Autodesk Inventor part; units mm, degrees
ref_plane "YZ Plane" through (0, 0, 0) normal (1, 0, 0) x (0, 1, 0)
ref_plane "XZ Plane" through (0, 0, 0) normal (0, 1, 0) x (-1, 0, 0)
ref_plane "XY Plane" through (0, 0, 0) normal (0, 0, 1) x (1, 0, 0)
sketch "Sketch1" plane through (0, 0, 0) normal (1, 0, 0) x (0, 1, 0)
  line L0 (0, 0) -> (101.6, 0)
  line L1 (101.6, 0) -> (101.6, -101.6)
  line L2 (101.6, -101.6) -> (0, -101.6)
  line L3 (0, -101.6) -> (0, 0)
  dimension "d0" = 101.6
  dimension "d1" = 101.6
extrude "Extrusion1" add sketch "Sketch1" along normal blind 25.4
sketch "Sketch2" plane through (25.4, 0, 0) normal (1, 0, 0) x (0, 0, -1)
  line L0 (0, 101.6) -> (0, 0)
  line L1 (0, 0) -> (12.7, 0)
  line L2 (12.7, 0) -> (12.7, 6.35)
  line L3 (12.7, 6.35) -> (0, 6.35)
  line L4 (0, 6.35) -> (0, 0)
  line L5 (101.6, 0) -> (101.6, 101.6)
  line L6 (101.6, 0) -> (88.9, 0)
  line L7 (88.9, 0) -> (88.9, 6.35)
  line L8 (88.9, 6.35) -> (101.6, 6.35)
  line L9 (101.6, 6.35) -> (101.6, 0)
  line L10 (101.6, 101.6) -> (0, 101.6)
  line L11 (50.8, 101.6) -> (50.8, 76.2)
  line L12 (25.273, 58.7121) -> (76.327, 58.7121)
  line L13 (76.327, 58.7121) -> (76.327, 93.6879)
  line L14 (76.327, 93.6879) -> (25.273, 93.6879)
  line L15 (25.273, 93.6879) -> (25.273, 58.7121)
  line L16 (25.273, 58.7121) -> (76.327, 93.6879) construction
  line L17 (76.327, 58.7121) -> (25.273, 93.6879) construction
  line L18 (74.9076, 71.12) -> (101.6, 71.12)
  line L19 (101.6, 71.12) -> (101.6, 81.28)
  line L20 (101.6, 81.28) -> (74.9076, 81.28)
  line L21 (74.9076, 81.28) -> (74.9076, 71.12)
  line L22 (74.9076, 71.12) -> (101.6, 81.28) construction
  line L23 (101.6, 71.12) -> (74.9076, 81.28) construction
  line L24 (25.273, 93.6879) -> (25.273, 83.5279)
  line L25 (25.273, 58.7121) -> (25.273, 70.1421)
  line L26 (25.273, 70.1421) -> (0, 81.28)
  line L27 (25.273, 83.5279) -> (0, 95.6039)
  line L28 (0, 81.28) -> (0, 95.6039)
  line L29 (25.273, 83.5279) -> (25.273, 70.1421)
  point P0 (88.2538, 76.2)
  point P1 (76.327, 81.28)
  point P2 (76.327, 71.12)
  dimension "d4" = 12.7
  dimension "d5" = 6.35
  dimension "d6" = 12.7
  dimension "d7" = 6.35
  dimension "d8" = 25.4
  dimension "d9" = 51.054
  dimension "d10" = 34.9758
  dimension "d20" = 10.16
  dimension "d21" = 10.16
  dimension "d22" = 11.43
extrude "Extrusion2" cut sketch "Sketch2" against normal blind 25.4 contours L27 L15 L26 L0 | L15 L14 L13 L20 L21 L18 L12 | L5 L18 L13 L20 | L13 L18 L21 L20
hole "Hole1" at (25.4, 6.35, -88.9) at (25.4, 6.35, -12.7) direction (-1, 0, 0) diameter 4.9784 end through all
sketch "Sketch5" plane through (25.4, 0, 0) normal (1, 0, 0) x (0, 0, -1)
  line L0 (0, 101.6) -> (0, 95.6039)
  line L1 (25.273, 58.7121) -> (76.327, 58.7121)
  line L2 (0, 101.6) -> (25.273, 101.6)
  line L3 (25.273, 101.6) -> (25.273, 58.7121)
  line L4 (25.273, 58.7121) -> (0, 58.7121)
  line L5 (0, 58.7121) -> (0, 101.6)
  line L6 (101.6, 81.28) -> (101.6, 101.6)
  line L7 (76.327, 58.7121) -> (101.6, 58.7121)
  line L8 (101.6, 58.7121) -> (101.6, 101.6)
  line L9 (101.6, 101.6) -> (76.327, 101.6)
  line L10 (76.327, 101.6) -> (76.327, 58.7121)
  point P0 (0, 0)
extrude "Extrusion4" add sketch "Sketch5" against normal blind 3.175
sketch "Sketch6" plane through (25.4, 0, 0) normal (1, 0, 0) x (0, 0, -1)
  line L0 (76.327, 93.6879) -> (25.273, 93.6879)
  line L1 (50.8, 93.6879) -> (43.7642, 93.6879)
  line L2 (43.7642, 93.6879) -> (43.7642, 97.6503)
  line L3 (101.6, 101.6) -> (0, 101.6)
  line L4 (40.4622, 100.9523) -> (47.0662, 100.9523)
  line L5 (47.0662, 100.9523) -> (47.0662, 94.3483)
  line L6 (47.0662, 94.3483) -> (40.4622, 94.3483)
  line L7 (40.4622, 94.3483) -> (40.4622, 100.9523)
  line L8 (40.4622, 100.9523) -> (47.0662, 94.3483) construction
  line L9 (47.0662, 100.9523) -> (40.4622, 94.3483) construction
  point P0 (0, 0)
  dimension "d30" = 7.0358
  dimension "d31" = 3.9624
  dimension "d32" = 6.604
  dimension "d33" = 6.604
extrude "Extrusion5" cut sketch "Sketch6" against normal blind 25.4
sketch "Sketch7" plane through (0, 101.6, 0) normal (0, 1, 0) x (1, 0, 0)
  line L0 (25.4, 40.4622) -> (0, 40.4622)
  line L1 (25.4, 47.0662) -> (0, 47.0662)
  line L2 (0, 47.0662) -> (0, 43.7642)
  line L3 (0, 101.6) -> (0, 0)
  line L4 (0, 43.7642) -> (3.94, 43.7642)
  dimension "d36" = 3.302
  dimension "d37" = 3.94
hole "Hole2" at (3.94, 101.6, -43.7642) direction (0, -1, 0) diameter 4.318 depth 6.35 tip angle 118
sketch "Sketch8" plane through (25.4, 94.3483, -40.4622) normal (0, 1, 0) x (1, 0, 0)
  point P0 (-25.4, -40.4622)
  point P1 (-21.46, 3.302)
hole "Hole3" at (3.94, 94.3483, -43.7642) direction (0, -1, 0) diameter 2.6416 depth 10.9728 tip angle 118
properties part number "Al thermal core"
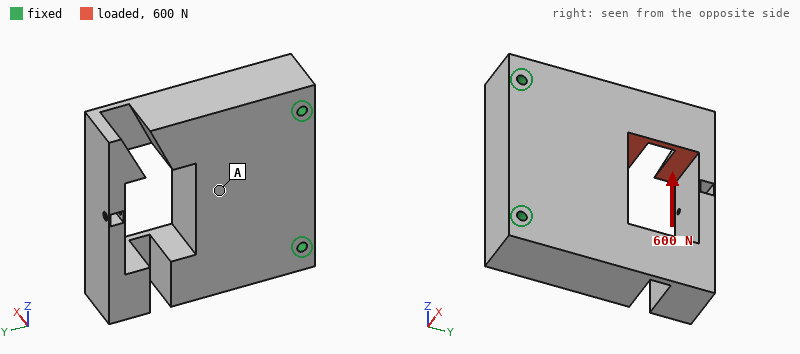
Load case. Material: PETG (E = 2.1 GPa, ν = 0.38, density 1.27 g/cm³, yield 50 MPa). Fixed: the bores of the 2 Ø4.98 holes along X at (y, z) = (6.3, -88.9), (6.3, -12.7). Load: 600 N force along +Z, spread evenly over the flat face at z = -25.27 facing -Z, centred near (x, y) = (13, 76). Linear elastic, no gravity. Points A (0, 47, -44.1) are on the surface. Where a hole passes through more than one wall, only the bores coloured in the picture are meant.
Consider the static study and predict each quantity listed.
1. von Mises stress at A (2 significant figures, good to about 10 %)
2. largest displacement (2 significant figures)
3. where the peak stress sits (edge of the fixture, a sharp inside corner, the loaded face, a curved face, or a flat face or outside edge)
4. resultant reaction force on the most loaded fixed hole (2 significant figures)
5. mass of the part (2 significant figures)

1.2 MPa
0.70 mm
a curved face
640 N
260 g
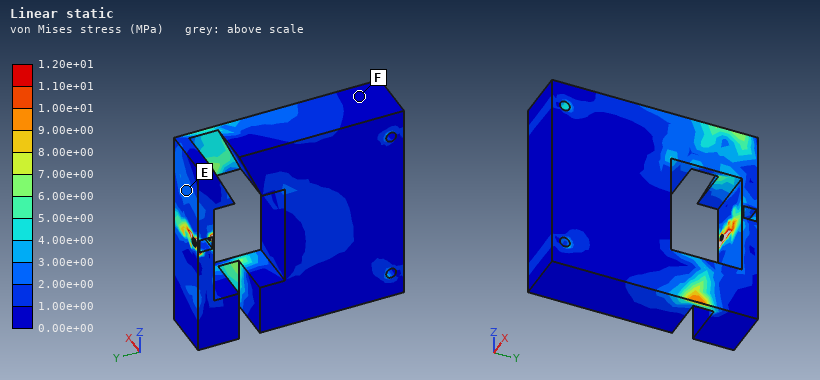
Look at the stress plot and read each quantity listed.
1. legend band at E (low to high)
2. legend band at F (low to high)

2.00e+00 to 3.00e+00 MPa
0.00e+00 to 1.00e+00 MPa
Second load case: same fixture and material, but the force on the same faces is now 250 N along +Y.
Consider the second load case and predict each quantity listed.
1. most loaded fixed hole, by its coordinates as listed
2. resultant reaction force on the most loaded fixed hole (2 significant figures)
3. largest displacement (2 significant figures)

(6.3, -12.7)
210 N
1.6 mm
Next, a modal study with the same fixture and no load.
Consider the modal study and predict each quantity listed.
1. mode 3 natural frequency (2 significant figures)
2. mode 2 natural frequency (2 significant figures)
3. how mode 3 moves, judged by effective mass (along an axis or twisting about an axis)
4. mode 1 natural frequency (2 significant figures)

650 Hz
530 Hz
along X
190 Hz
